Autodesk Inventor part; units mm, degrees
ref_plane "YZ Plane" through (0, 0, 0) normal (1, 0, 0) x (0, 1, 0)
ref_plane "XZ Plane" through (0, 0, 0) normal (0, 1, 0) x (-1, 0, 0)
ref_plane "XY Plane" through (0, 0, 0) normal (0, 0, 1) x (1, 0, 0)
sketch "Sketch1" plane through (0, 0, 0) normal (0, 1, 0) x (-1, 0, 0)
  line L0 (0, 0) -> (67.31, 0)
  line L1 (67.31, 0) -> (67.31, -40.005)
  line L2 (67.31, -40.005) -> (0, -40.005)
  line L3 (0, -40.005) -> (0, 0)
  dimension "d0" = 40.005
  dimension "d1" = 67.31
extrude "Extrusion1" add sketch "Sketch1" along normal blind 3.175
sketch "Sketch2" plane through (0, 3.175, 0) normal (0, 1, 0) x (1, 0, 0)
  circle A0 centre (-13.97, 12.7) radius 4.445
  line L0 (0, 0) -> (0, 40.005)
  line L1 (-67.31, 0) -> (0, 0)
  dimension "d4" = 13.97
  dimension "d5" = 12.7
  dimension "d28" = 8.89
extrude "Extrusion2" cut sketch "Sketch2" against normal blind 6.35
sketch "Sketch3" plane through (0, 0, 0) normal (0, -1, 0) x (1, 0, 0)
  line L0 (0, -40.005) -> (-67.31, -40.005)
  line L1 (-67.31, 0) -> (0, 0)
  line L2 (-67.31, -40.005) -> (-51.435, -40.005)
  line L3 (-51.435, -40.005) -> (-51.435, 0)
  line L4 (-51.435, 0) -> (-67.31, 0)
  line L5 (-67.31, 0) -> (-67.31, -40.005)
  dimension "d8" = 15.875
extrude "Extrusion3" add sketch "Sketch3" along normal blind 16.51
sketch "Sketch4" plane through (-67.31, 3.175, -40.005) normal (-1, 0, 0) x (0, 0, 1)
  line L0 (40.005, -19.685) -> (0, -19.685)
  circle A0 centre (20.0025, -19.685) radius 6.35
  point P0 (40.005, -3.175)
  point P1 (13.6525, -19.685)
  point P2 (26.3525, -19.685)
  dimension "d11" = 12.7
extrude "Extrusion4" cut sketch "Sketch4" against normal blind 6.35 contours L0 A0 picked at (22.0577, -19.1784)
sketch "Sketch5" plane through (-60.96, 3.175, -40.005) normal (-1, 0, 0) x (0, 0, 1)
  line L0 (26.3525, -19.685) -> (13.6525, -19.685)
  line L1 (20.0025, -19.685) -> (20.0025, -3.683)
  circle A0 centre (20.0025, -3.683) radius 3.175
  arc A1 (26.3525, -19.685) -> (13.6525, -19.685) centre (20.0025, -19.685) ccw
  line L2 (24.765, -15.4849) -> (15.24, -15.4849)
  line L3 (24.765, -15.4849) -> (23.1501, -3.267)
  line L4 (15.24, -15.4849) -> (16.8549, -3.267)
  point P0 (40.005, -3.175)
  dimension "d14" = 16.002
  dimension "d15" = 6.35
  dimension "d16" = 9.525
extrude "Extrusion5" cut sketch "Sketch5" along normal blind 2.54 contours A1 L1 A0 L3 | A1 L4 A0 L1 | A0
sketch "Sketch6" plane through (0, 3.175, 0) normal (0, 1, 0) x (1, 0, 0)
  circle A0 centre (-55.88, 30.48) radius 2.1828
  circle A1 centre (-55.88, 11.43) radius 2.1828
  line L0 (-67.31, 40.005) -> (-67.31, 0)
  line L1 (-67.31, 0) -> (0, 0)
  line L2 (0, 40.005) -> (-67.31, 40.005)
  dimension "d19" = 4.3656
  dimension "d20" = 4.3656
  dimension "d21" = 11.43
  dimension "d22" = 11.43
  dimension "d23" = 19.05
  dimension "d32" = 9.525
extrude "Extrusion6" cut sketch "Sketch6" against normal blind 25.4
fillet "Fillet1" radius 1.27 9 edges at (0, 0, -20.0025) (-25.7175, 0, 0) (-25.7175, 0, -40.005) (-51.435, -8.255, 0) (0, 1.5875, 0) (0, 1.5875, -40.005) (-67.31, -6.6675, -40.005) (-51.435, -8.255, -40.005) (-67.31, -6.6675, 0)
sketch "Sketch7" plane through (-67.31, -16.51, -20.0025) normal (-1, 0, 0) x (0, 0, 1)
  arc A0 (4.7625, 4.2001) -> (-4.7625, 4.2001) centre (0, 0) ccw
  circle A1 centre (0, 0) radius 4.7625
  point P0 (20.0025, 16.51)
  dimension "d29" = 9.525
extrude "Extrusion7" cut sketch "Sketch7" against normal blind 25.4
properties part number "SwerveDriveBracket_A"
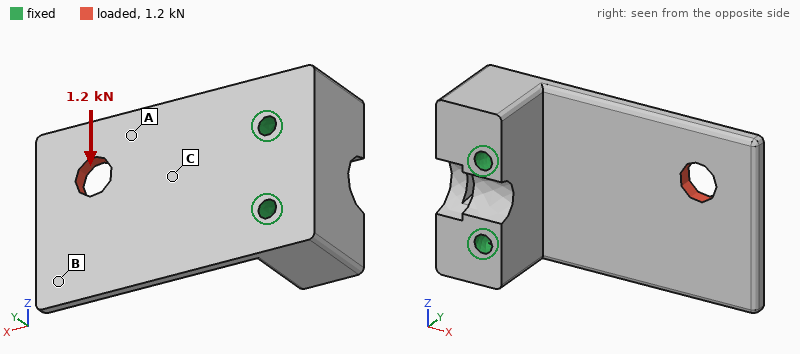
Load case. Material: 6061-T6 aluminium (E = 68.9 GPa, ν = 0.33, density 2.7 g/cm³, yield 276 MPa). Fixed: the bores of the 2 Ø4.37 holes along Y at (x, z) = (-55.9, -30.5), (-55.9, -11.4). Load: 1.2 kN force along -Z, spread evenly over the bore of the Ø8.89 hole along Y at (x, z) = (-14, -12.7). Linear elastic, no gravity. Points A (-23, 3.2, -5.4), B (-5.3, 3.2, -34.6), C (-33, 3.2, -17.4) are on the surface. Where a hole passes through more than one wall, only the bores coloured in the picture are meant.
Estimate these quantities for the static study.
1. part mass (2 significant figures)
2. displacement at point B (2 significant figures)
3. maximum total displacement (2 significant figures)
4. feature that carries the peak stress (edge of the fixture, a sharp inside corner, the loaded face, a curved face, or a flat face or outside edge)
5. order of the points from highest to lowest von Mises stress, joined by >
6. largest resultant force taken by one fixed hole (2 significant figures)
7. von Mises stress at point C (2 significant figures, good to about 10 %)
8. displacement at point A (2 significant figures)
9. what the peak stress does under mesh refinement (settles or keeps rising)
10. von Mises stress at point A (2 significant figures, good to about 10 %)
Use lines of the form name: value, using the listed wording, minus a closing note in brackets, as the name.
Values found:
part mass: 46 g
displacement at point B: 60 µm
maximum total displacement: 68 µm
feature that carries the peak stress: edge of the fixture
order of the points from highest to lowest von Mises stress, joined by >: C > A > B
largest resultant force taken by one fixed hole: 2.2 kN
von Mises stress at point C: 26 MPa
displacement at point A: 39 µm
what the peak stress does under mesh refinement: keeps rising
von Mises stress at point A: 15 MPa
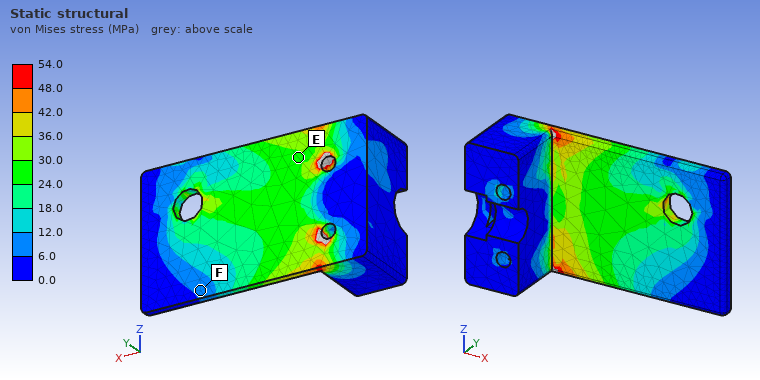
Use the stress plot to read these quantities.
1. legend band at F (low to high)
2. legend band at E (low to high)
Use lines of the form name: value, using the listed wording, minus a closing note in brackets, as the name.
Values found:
legend band at F: 6.0 to 12.0 MPa
legend band at E: 24.0 to 30.0 MPa
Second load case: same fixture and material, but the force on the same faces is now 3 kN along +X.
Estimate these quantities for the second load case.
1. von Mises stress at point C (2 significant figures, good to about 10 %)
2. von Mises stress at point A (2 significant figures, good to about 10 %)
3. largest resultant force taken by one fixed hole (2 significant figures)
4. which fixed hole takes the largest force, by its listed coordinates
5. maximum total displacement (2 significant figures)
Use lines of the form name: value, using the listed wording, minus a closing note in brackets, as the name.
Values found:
von Mises stress at point C: 31 MPa
von Mises stress at point A: 43 MPa
largest resultant force taken by one fixed hole: 2.6 kN
which fixed hole takes the largest force, by its listed coordinates: (-55.9, -11.4)
maximum total displacement: 45 µm
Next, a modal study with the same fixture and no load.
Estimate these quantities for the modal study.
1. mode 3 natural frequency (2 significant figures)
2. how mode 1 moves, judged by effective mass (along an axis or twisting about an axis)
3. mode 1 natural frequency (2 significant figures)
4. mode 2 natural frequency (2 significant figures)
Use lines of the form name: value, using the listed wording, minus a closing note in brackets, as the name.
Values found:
mode 3 natural frequency: 5700 Hz
how mode 1 moves, judged by effective mass: along Y
mode 1 natural frequency: 970 Hz
mode 2 natural frequency: 2800 Hz
